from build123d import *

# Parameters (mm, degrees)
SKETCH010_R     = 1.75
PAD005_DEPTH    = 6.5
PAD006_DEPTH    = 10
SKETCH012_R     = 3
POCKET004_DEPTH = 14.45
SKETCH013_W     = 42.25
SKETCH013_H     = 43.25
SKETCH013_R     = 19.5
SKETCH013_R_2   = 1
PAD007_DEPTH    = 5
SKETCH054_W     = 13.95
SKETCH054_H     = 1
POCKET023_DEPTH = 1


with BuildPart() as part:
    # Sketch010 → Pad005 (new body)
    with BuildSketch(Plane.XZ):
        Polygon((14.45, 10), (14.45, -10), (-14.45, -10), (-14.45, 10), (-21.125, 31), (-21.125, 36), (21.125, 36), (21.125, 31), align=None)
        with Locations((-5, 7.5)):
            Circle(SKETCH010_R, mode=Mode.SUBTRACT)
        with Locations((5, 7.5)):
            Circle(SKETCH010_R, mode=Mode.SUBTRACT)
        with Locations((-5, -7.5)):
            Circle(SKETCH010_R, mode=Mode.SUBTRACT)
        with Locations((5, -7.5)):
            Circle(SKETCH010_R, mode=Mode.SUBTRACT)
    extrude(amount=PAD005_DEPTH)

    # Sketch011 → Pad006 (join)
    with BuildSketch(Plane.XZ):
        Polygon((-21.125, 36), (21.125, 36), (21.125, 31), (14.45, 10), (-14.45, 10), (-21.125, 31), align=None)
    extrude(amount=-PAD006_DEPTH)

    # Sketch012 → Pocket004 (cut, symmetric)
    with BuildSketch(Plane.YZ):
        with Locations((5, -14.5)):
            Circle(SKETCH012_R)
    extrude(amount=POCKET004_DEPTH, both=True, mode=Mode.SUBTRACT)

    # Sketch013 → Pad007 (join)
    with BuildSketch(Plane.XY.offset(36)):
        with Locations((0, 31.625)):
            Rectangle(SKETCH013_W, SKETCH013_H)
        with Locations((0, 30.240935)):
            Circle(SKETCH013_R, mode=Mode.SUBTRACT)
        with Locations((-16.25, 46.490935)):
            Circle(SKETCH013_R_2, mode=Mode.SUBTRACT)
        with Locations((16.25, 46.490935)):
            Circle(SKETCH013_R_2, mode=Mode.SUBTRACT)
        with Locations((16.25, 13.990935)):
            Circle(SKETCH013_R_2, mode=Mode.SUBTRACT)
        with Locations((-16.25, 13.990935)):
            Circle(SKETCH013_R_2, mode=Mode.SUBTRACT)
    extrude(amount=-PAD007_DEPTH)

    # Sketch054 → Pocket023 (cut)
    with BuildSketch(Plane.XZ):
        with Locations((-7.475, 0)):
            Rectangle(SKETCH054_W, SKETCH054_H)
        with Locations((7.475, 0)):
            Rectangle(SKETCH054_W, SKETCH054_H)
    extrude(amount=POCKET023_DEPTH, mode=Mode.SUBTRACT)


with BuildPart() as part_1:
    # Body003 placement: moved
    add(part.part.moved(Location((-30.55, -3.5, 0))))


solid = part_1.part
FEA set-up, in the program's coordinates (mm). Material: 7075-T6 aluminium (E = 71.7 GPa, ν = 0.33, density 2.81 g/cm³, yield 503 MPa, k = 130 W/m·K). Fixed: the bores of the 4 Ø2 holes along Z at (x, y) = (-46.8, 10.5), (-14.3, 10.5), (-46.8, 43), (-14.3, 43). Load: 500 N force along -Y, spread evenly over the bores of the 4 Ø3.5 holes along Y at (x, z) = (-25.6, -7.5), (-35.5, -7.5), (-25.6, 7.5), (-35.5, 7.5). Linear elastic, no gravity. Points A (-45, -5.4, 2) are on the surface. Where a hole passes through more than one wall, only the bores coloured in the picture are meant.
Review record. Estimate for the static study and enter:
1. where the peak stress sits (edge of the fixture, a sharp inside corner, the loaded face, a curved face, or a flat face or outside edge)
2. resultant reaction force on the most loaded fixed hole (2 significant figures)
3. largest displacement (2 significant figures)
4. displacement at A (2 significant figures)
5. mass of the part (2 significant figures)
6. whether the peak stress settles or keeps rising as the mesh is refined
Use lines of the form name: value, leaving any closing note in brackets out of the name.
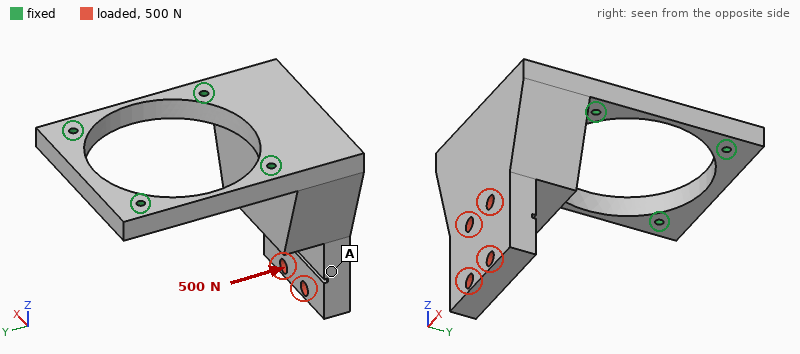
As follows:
where the peak stress sits: edge of the fixture
resultant reaction force on the most loaded fixed hole: 260 N
largest displacement: 0.39 mm
displacement at A: 0.27 mm
mass of the part: 63 g
whether the peak stress settles or keeps rising as the mesh is refined: keeps rising
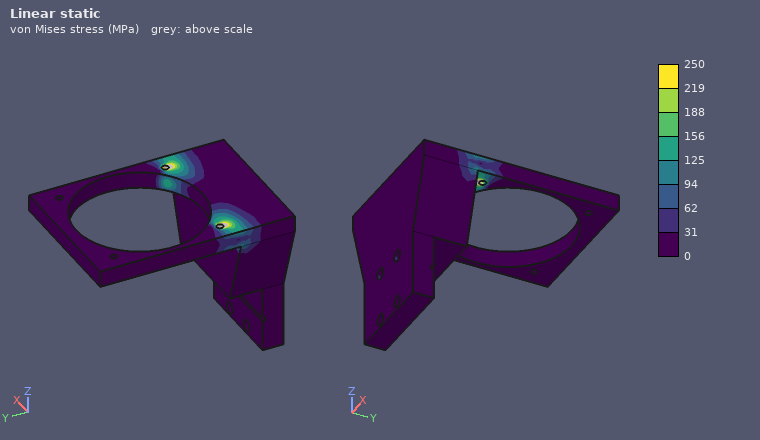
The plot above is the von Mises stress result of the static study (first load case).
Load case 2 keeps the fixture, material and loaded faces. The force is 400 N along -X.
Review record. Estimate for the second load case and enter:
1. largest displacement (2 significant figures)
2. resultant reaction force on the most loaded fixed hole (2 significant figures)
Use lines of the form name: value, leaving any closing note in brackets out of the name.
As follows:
largest displacement: 17 µm
resultant reaction force on the most loaded fixed hole: 490 N
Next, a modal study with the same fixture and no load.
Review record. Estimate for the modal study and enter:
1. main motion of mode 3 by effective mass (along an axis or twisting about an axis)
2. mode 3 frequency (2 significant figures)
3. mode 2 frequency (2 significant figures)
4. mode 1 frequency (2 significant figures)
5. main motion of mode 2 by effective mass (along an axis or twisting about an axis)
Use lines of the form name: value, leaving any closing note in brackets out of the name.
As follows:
main motion of mode 3 by effective mass: along Z
mode 3 frequency: 9200 Hz
mode 2 frequency: 6500 Hz
mode 1 frequency: 1500 Hz
main motion of mode 2 by effective mass: along X
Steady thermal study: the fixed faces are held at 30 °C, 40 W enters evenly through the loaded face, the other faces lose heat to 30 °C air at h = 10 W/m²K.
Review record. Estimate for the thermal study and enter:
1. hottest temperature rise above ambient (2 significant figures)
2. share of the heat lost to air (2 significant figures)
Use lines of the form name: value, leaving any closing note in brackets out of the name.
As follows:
hottest temperature rise above ambient: 60 K
share of the heat lost to air: 4.4 %
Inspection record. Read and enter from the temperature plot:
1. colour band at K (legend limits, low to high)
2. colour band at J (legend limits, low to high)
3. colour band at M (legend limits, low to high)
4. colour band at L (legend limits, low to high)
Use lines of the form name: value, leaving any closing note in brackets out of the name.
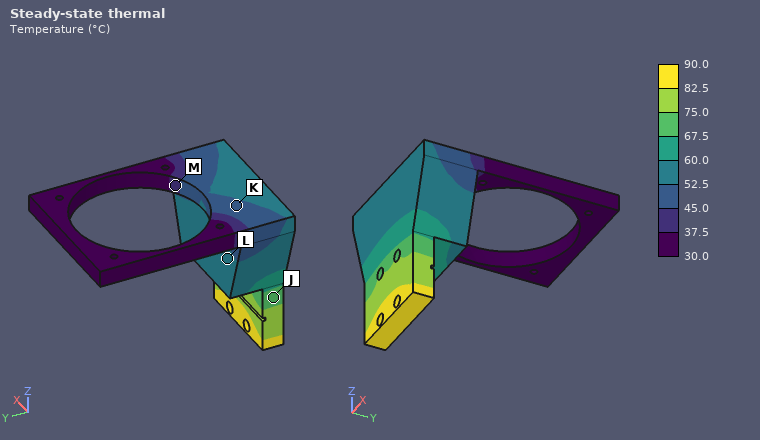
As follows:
colour band at K: 45.0 to 52.5 °C
colour band at J: 67.5 to 75.0 °C
colour band at M: 37.5 to 45.0 °C
colour band at L: 52.5 to 60.0 °C
